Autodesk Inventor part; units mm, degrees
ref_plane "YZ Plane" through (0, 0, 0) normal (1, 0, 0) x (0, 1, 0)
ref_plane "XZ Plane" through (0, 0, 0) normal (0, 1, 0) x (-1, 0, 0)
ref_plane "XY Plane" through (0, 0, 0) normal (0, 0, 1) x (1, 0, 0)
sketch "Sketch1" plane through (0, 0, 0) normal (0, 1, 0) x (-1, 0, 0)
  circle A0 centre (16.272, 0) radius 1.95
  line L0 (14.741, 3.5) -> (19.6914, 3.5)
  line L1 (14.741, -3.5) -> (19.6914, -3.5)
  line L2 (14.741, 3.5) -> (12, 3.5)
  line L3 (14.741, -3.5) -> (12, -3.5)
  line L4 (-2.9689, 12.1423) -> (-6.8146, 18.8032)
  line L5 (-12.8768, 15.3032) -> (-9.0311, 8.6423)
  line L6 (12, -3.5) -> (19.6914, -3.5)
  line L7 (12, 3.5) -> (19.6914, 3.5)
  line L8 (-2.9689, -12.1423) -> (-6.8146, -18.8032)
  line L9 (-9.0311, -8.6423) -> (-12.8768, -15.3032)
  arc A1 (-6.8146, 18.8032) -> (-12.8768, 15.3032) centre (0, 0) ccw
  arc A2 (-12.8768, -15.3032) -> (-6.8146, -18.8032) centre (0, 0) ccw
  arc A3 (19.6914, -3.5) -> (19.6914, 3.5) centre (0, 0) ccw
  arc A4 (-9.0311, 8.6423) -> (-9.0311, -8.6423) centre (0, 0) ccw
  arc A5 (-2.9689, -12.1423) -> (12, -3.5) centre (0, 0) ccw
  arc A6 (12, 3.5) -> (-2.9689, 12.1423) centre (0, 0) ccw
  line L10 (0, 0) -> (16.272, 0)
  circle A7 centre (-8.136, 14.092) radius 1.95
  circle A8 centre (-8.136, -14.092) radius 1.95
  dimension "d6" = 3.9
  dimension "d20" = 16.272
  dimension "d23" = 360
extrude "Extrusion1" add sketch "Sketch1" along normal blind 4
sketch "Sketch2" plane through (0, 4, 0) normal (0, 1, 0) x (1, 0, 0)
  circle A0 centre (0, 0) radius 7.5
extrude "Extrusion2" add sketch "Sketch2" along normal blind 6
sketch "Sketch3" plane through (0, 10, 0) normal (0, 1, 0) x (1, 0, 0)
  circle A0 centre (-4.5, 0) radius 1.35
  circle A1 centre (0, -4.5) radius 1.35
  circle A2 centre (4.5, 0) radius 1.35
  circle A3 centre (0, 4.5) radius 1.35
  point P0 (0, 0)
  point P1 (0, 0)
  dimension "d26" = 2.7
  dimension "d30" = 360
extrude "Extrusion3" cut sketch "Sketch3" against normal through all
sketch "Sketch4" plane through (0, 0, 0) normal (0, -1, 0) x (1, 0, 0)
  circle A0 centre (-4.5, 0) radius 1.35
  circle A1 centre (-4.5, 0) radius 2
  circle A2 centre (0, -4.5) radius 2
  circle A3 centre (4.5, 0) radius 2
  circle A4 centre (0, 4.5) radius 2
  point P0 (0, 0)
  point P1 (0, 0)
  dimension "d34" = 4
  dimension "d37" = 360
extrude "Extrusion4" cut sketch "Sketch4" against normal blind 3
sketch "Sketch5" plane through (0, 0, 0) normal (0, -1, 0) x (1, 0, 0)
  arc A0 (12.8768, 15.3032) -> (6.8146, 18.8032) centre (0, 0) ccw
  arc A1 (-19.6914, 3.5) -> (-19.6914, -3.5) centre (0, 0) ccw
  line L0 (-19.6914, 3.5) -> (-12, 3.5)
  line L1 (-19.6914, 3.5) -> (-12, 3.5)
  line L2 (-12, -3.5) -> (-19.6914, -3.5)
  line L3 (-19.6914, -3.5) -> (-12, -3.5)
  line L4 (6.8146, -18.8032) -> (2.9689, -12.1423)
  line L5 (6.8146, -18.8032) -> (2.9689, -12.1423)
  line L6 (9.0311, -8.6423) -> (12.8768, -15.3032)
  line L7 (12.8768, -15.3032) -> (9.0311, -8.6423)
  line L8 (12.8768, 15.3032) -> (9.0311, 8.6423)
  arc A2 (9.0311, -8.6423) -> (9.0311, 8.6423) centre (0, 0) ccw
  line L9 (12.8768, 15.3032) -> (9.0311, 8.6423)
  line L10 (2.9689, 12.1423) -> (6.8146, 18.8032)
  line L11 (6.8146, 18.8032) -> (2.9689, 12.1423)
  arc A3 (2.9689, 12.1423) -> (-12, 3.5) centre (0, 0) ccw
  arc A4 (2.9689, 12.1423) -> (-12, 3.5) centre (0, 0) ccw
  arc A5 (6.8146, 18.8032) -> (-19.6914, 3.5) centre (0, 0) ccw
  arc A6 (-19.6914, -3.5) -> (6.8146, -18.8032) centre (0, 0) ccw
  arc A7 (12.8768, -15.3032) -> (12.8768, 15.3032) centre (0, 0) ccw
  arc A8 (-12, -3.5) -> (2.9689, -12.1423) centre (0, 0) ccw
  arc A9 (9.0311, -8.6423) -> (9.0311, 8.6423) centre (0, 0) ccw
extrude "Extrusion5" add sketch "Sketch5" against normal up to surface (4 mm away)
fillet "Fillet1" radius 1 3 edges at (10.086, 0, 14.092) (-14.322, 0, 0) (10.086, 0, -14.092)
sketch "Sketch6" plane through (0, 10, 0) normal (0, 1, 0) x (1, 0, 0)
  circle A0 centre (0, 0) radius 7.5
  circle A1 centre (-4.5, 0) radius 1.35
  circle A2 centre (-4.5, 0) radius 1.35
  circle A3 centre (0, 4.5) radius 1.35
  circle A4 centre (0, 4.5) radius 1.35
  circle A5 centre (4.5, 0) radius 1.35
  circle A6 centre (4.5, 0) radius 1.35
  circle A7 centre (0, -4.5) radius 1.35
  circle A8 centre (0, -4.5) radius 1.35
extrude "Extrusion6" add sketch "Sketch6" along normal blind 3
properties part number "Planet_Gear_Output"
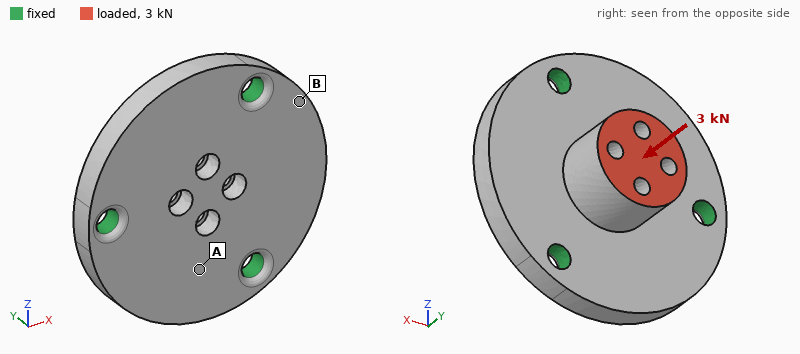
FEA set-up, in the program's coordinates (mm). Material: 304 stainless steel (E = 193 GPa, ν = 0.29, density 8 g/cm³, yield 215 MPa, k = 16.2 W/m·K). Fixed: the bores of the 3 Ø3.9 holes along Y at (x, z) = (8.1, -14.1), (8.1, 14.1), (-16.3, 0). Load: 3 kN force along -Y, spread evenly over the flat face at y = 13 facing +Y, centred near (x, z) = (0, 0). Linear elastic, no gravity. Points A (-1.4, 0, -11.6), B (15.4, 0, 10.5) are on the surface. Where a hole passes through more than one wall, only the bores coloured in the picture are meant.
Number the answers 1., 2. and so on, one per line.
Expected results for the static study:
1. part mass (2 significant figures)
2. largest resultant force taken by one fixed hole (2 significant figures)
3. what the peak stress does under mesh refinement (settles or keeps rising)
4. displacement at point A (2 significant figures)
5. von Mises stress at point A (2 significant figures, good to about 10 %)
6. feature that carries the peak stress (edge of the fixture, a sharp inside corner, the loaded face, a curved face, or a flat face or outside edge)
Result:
1. 49 g
2. 1.0 kN
3. keeps rising
4. 6.7 µm
5. 46 MPa
6. edge of the fixture
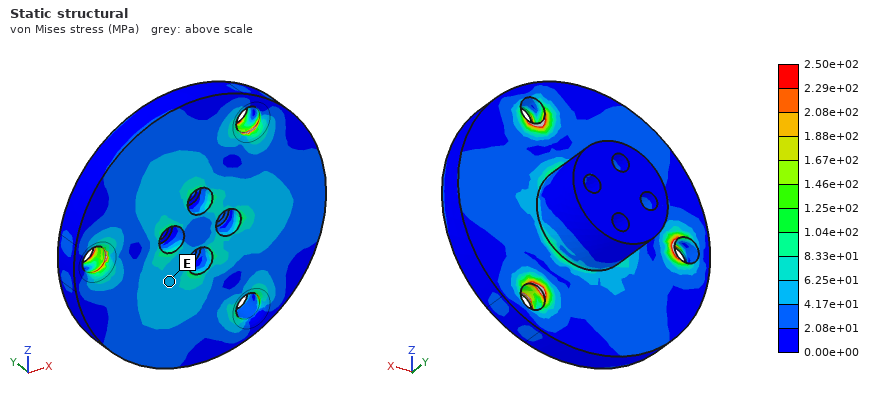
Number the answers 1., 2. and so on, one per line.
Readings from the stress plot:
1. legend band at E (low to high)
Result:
1. 4.17e+01 to 6.25e+01 MPa
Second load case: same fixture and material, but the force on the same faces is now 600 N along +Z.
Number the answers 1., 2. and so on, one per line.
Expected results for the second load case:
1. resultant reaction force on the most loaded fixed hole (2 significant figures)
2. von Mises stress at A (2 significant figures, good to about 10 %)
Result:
1. 320 N
2. 13 MPa
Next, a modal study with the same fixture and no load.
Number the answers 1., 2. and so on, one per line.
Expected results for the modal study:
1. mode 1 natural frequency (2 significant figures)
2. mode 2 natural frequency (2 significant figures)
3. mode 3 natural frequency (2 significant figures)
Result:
1. 16 kHz
2. 16 kHz
3. 16 kHz
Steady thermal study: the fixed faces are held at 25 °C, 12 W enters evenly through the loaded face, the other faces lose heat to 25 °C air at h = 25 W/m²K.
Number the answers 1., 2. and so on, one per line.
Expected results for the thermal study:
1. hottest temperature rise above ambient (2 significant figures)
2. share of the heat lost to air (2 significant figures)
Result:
1. 83 K
2. 20 %
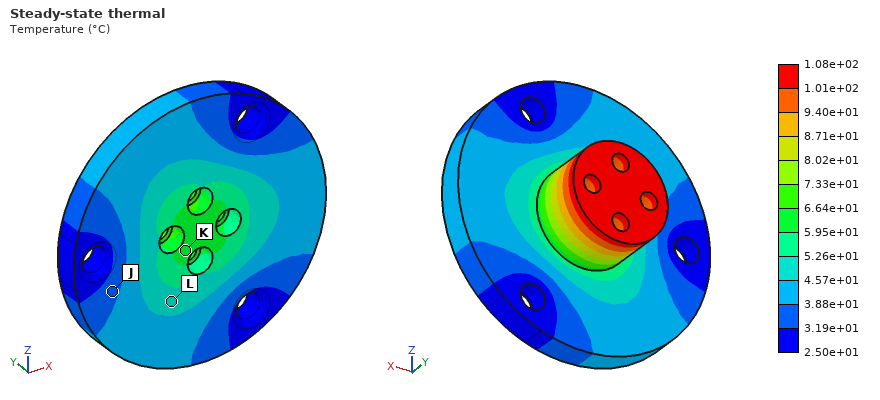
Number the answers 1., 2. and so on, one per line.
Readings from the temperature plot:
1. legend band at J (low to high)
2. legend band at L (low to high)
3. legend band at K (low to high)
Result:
1. 3.19e+01 to 3.88e+01 °C
2. 4.57e+01 to 5.26e+01 °C
3. 5.95e+01 to 6.64e+01 °C
